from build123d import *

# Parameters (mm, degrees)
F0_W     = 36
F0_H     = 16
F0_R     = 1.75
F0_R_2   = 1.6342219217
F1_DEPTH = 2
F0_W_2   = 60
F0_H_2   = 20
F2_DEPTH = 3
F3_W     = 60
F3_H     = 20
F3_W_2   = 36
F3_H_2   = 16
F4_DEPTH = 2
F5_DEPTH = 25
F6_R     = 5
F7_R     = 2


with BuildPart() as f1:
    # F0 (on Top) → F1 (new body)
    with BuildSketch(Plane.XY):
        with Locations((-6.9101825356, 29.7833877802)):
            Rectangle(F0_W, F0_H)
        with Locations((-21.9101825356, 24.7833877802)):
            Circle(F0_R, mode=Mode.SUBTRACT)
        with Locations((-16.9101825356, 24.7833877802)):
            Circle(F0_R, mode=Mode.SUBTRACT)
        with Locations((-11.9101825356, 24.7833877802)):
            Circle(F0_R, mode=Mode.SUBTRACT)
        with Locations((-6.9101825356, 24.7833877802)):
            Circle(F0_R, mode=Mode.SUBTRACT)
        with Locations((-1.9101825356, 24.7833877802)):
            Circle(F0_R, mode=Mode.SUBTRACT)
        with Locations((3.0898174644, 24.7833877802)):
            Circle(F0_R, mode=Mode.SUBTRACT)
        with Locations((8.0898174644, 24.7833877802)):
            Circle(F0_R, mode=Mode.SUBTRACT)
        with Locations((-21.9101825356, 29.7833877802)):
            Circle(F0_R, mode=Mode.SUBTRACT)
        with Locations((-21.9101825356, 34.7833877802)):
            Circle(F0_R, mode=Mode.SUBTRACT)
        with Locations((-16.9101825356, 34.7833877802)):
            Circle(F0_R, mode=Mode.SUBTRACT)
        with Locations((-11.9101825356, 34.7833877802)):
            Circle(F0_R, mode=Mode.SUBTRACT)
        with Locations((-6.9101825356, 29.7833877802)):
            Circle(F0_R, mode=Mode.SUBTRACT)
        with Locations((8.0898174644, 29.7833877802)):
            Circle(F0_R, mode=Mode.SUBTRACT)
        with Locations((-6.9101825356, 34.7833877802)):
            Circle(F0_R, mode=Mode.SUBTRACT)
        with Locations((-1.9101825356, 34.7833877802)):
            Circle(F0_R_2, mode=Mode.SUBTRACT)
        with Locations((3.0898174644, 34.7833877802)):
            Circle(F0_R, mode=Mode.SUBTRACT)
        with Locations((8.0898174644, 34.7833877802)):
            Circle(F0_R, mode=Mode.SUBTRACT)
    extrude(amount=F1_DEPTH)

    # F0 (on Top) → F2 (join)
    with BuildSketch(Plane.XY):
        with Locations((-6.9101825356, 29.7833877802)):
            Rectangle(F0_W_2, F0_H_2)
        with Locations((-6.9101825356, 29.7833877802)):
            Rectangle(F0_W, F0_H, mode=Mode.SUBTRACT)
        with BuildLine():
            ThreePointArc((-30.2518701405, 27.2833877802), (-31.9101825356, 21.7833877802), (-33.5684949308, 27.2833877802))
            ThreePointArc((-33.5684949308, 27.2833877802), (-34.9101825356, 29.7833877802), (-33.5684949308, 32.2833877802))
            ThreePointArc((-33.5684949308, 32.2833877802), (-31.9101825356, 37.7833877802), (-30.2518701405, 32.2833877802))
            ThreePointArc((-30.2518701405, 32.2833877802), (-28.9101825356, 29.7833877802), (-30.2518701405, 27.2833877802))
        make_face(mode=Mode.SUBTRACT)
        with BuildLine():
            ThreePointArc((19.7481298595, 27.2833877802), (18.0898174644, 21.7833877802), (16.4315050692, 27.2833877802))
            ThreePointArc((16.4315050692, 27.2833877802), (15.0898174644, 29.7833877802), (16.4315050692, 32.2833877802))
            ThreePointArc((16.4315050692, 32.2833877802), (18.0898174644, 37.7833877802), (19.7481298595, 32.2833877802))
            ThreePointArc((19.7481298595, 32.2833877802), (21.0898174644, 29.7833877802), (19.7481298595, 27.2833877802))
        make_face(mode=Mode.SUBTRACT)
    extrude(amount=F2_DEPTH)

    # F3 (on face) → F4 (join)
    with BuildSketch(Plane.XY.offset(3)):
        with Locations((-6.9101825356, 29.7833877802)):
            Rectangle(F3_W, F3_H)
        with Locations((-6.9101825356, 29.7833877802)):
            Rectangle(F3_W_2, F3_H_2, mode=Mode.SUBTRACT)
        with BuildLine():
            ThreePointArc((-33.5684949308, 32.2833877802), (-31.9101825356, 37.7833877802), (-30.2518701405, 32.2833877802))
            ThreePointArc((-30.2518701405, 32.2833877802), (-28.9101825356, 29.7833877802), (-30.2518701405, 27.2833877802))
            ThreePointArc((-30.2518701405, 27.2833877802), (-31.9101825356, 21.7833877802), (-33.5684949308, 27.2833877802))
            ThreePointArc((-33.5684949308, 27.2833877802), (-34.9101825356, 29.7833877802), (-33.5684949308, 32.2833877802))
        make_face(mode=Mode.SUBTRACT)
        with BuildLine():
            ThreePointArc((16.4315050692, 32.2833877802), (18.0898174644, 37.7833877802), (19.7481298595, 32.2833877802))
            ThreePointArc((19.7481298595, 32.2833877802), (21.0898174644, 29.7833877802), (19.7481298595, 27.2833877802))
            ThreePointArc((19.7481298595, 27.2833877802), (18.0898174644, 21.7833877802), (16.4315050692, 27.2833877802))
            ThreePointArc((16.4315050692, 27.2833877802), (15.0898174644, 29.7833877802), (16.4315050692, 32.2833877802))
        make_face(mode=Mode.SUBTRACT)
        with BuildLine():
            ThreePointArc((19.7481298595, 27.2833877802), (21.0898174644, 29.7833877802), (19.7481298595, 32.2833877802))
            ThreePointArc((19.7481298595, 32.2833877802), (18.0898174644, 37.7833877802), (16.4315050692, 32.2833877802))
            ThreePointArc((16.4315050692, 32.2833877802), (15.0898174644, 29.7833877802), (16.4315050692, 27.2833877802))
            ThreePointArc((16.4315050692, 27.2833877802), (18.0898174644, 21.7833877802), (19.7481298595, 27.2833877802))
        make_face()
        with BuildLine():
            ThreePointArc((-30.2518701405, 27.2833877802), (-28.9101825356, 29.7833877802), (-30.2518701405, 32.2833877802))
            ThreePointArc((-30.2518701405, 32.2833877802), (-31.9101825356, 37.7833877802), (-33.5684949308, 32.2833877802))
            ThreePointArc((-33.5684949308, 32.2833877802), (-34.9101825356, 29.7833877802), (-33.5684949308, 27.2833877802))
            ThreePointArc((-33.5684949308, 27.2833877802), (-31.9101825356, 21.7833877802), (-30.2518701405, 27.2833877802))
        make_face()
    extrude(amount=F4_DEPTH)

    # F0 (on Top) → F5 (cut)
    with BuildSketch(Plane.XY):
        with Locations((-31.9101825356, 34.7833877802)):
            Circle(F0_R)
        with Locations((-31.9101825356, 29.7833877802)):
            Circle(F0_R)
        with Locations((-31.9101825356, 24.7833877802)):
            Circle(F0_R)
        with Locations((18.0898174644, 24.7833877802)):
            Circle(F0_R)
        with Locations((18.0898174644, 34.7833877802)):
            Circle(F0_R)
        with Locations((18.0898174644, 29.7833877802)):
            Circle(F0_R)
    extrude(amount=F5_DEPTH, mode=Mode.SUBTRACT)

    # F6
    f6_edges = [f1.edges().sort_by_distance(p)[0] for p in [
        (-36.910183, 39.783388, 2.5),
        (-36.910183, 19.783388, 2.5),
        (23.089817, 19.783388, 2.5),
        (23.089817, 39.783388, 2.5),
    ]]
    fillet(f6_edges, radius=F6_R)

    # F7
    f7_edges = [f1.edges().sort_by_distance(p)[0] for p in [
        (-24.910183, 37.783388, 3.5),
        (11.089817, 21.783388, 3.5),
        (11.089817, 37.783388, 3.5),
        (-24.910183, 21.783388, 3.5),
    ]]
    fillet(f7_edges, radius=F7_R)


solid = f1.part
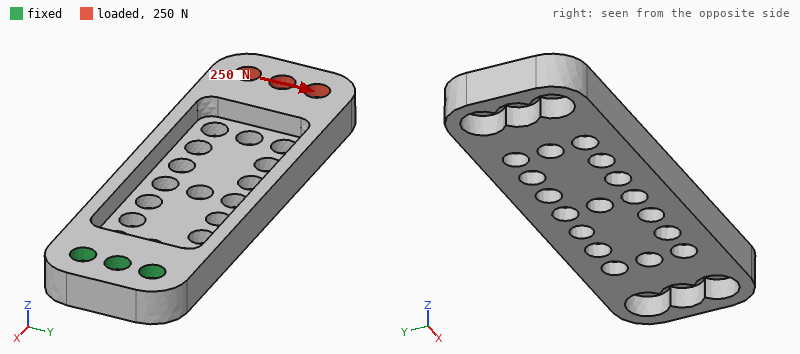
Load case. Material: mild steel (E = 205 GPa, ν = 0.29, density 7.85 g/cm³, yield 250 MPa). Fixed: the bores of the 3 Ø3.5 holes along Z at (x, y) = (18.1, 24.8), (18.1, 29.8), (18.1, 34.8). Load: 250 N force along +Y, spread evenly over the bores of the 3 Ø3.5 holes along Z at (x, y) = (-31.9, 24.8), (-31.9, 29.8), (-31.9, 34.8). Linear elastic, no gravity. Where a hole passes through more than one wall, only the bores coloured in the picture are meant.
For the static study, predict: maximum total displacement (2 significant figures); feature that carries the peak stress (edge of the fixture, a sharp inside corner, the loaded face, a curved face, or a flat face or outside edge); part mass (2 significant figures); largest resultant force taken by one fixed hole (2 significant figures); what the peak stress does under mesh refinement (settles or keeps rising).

95 µm
edge of the fixture
26 g
930 N
keeps rising
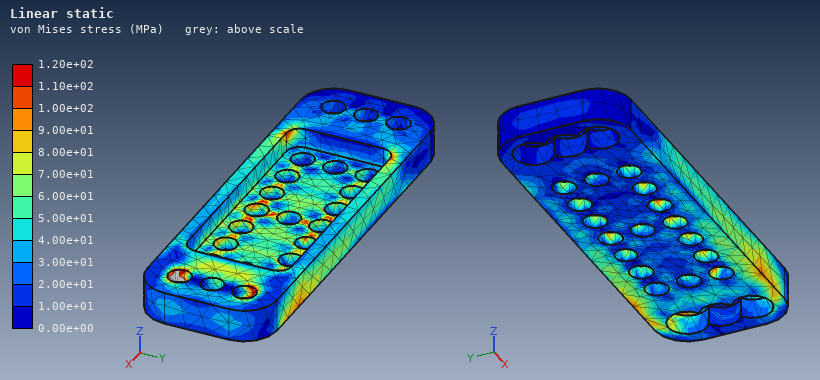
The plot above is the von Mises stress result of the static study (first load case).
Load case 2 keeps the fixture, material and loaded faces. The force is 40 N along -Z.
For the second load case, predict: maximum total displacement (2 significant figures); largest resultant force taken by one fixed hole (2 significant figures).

0.15 mm
66 N
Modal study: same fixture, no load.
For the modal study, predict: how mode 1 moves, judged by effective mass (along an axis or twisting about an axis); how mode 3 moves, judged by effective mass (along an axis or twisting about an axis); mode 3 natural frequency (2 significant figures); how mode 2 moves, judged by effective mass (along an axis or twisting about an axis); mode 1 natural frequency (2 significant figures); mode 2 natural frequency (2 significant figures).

along Z
along Y
4700 Hz
along Y
970 Hz
2800 Hz
